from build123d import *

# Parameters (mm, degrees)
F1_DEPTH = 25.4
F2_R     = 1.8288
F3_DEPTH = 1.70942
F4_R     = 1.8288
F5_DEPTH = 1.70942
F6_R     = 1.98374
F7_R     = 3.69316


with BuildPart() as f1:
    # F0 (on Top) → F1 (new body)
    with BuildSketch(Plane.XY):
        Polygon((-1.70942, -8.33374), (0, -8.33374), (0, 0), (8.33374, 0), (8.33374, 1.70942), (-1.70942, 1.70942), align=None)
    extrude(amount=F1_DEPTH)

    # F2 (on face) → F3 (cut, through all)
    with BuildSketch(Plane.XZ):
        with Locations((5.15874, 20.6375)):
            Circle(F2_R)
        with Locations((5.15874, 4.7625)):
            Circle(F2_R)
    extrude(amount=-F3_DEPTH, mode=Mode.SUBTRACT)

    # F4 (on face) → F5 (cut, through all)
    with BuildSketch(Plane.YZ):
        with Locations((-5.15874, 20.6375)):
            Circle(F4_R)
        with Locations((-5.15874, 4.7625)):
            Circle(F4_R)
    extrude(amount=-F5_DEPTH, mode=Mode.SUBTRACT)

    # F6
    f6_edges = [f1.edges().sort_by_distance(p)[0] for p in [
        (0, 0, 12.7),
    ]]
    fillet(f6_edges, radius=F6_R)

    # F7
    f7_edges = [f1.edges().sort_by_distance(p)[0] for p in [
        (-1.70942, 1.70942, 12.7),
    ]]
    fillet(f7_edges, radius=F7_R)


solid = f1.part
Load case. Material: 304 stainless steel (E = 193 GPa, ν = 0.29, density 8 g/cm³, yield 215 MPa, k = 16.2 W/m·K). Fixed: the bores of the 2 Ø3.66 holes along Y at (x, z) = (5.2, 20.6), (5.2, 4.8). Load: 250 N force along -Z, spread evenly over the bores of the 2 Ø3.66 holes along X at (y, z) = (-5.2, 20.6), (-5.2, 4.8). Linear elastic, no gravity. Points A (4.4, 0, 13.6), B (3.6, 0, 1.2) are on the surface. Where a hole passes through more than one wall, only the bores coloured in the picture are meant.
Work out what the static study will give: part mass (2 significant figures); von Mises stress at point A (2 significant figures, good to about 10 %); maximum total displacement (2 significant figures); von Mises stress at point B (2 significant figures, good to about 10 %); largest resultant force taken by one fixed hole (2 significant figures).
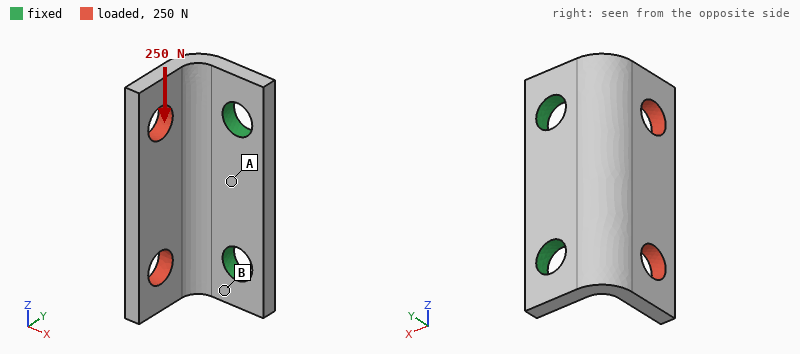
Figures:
5.4 g
12 MPa
8.5 µm
28 MPa
170 N
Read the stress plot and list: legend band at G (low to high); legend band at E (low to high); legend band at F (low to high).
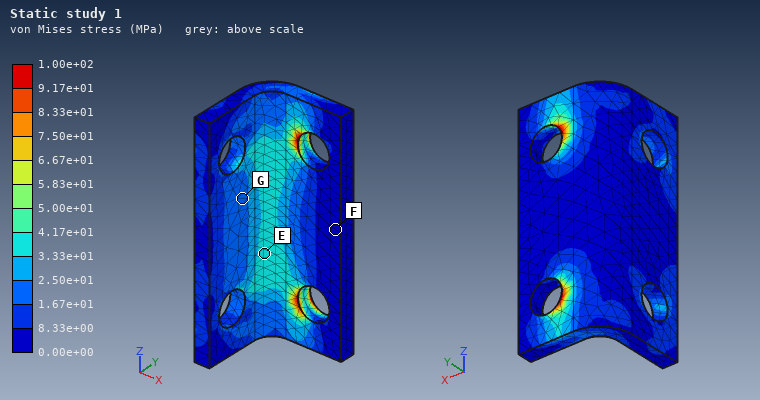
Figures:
1.67e+01 to 2.50e+01 MPa
3.33e+01 to 4.17e+01 MPa
0.00e+00 to 8.33e+00 MPa
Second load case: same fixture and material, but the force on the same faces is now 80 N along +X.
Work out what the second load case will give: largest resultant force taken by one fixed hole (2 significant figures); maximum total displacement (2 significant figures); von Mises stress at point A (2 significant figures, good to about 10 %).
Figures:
40 N
15 µm
14 MPa
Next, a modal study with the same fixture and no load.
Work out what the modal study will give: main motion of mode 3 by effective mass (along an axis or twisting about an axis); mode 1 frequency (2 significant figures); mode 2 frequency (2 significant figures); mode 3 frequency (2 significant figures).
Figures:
along Y
9500 Hz
14 kHz
27 kHz
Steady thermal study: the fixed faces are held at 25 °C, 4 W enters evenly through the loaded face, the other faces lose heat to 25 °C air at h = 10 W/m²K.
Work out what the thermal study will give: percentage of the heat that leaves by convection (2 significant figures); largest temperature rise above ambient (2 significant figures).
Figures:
7.1 %
77 K
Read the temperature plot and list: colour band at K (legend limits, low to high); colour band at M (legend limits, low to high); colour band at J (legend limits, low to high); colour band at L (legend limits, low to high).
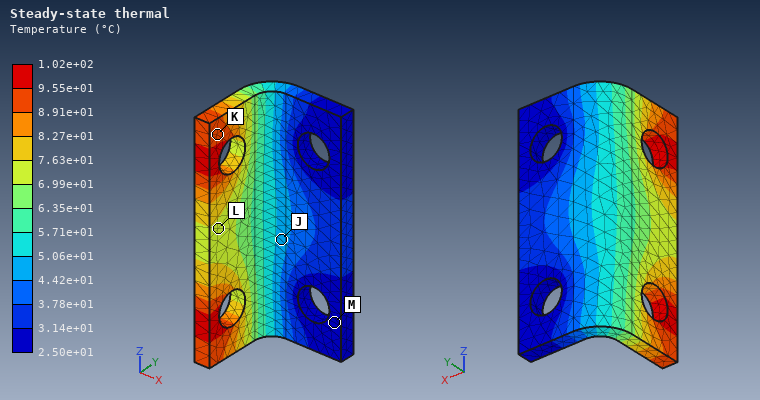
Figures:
8.91e+01 to 9.55e+01 °C
2.50e+01 to 3.14e+01 °C
4.42e+01 to 5.06e+01 °C
6.99e+01 to 7.63e+01 °C
